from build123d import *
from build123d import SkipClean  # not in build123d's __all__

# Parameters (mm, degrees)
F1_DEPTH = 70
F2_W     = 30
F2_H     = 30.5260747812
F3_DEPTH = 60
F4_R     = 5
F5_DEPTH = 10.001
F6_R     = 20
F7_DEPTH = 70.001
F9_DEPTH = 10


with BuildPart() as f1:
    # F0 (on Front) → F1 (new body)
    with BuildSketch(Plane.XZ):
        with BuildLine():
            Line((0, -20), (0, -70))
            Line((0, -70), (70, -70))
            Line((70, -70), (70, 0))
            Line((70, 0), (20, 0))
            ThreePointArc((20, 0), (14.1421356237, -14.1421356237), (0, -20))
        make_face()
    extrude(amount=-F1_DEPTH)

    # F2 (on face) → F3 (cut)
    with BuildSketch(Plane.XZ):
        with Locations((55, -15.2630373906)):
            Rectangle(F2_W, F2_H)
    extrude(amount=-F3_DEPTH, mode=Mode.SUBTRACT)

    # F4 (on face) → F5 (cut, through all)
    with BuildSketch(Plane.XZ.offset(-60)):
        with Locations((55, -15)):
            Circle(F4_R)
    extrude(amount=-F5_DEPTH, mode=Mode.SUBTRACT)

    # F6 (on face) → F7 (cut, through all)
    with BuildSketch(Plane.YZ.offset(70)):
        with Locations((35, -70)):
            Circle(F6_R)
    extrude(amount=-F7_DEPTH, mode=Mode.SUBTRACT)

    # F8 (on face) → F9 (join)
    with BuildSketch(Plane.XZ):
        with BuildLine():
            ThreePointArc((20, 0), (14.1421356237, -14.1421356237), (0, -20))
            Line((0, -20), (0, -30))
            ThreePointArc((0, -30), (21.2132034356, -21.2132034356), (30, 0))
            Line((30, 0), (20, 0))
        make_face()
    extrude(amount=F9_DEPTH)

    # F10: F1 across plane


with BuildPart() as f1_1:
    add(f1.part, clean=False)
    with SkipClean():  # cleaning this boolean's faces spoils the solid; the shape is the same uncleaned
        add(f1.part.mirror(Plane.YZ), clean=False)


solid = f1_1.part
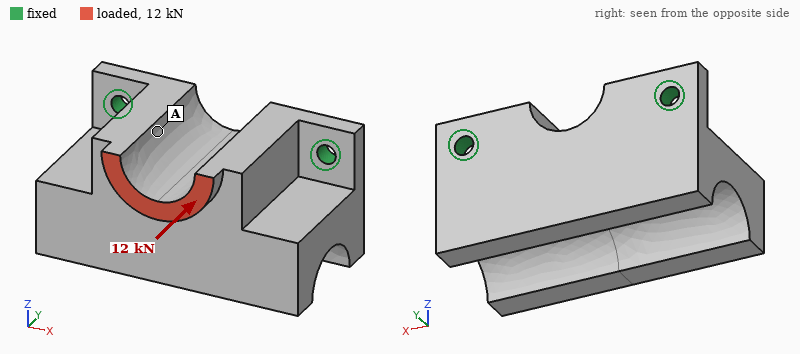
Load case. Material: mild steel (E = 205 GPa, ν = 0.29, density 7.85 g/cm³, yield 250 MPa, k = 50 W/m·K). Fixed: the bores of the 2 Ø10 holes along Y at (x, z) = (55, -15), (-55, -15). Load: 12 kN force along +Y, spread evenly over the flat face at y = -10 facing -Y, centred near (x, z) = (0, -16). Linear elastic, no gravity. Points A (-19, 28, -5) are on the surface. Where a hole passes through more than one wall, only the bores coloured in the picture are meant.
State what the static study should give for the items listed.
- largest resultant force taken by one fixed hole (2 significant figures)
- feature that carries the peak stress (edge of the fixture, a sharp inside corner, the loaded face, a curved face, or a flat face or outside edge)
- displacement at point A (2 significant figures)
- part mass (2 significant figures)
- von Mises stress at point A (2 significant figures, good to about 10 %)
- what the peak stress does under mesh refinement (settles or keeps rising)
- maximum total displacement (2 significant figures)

6.3 kN
edge of the fixture
13 µm
3.5 kg
10 MPa
keeps rising
23 µm
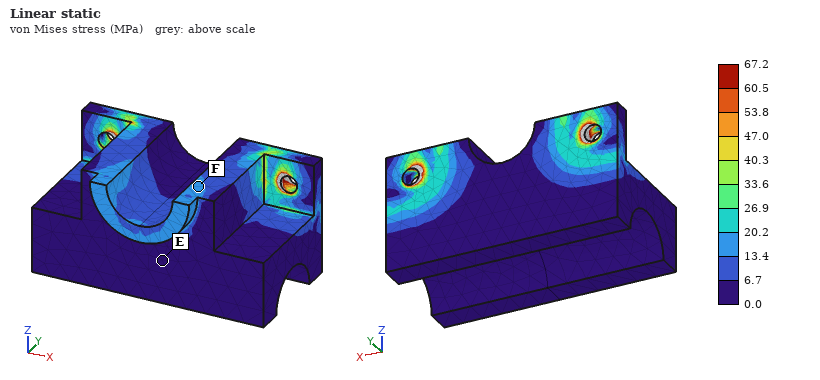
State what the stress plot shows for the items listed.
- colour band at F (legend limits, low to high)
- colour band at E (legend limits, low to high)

13.4 to 20.2 MPa
0.0 to 6.7 MPa
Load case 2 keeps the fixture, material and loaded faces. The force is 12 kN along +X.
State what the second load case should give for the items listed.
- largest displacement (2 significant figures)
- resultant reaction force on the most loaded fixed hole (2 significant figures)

39 µm
11 kN
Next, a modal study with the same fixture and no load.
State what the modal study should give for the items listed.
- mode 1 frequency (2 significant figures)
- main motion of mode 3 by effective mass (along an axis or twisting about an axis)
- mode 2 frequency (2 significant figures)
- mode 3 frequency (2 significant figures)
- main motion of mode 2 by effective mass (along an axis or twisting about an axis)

790 Hz
along Y
3200 Hz
3800 Hz
along X
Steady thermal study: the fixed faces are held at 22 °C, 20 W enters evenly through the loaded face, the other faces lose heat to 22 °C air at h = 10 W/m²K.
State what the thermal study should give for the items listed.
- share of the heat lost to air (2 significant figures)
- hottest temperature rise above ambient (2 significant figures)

21 %
20 K
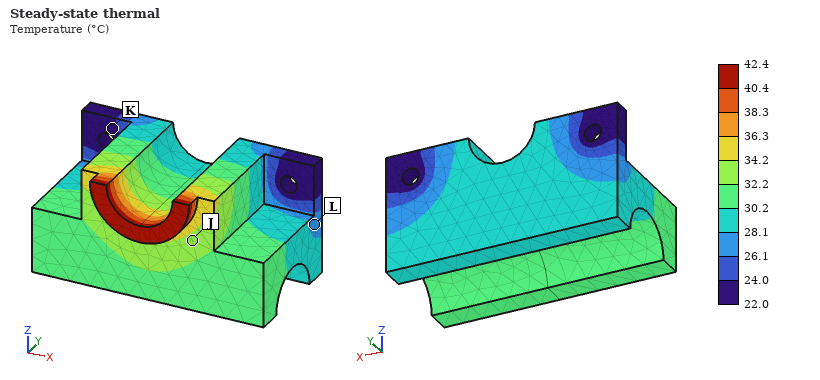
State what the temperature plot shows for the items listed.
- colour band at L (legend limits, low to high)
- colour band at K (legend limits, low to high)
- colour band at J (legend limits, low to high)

26.1 to 28.1 °C
22.0 to 24.0 °C
32.2 to 34.2 °C
